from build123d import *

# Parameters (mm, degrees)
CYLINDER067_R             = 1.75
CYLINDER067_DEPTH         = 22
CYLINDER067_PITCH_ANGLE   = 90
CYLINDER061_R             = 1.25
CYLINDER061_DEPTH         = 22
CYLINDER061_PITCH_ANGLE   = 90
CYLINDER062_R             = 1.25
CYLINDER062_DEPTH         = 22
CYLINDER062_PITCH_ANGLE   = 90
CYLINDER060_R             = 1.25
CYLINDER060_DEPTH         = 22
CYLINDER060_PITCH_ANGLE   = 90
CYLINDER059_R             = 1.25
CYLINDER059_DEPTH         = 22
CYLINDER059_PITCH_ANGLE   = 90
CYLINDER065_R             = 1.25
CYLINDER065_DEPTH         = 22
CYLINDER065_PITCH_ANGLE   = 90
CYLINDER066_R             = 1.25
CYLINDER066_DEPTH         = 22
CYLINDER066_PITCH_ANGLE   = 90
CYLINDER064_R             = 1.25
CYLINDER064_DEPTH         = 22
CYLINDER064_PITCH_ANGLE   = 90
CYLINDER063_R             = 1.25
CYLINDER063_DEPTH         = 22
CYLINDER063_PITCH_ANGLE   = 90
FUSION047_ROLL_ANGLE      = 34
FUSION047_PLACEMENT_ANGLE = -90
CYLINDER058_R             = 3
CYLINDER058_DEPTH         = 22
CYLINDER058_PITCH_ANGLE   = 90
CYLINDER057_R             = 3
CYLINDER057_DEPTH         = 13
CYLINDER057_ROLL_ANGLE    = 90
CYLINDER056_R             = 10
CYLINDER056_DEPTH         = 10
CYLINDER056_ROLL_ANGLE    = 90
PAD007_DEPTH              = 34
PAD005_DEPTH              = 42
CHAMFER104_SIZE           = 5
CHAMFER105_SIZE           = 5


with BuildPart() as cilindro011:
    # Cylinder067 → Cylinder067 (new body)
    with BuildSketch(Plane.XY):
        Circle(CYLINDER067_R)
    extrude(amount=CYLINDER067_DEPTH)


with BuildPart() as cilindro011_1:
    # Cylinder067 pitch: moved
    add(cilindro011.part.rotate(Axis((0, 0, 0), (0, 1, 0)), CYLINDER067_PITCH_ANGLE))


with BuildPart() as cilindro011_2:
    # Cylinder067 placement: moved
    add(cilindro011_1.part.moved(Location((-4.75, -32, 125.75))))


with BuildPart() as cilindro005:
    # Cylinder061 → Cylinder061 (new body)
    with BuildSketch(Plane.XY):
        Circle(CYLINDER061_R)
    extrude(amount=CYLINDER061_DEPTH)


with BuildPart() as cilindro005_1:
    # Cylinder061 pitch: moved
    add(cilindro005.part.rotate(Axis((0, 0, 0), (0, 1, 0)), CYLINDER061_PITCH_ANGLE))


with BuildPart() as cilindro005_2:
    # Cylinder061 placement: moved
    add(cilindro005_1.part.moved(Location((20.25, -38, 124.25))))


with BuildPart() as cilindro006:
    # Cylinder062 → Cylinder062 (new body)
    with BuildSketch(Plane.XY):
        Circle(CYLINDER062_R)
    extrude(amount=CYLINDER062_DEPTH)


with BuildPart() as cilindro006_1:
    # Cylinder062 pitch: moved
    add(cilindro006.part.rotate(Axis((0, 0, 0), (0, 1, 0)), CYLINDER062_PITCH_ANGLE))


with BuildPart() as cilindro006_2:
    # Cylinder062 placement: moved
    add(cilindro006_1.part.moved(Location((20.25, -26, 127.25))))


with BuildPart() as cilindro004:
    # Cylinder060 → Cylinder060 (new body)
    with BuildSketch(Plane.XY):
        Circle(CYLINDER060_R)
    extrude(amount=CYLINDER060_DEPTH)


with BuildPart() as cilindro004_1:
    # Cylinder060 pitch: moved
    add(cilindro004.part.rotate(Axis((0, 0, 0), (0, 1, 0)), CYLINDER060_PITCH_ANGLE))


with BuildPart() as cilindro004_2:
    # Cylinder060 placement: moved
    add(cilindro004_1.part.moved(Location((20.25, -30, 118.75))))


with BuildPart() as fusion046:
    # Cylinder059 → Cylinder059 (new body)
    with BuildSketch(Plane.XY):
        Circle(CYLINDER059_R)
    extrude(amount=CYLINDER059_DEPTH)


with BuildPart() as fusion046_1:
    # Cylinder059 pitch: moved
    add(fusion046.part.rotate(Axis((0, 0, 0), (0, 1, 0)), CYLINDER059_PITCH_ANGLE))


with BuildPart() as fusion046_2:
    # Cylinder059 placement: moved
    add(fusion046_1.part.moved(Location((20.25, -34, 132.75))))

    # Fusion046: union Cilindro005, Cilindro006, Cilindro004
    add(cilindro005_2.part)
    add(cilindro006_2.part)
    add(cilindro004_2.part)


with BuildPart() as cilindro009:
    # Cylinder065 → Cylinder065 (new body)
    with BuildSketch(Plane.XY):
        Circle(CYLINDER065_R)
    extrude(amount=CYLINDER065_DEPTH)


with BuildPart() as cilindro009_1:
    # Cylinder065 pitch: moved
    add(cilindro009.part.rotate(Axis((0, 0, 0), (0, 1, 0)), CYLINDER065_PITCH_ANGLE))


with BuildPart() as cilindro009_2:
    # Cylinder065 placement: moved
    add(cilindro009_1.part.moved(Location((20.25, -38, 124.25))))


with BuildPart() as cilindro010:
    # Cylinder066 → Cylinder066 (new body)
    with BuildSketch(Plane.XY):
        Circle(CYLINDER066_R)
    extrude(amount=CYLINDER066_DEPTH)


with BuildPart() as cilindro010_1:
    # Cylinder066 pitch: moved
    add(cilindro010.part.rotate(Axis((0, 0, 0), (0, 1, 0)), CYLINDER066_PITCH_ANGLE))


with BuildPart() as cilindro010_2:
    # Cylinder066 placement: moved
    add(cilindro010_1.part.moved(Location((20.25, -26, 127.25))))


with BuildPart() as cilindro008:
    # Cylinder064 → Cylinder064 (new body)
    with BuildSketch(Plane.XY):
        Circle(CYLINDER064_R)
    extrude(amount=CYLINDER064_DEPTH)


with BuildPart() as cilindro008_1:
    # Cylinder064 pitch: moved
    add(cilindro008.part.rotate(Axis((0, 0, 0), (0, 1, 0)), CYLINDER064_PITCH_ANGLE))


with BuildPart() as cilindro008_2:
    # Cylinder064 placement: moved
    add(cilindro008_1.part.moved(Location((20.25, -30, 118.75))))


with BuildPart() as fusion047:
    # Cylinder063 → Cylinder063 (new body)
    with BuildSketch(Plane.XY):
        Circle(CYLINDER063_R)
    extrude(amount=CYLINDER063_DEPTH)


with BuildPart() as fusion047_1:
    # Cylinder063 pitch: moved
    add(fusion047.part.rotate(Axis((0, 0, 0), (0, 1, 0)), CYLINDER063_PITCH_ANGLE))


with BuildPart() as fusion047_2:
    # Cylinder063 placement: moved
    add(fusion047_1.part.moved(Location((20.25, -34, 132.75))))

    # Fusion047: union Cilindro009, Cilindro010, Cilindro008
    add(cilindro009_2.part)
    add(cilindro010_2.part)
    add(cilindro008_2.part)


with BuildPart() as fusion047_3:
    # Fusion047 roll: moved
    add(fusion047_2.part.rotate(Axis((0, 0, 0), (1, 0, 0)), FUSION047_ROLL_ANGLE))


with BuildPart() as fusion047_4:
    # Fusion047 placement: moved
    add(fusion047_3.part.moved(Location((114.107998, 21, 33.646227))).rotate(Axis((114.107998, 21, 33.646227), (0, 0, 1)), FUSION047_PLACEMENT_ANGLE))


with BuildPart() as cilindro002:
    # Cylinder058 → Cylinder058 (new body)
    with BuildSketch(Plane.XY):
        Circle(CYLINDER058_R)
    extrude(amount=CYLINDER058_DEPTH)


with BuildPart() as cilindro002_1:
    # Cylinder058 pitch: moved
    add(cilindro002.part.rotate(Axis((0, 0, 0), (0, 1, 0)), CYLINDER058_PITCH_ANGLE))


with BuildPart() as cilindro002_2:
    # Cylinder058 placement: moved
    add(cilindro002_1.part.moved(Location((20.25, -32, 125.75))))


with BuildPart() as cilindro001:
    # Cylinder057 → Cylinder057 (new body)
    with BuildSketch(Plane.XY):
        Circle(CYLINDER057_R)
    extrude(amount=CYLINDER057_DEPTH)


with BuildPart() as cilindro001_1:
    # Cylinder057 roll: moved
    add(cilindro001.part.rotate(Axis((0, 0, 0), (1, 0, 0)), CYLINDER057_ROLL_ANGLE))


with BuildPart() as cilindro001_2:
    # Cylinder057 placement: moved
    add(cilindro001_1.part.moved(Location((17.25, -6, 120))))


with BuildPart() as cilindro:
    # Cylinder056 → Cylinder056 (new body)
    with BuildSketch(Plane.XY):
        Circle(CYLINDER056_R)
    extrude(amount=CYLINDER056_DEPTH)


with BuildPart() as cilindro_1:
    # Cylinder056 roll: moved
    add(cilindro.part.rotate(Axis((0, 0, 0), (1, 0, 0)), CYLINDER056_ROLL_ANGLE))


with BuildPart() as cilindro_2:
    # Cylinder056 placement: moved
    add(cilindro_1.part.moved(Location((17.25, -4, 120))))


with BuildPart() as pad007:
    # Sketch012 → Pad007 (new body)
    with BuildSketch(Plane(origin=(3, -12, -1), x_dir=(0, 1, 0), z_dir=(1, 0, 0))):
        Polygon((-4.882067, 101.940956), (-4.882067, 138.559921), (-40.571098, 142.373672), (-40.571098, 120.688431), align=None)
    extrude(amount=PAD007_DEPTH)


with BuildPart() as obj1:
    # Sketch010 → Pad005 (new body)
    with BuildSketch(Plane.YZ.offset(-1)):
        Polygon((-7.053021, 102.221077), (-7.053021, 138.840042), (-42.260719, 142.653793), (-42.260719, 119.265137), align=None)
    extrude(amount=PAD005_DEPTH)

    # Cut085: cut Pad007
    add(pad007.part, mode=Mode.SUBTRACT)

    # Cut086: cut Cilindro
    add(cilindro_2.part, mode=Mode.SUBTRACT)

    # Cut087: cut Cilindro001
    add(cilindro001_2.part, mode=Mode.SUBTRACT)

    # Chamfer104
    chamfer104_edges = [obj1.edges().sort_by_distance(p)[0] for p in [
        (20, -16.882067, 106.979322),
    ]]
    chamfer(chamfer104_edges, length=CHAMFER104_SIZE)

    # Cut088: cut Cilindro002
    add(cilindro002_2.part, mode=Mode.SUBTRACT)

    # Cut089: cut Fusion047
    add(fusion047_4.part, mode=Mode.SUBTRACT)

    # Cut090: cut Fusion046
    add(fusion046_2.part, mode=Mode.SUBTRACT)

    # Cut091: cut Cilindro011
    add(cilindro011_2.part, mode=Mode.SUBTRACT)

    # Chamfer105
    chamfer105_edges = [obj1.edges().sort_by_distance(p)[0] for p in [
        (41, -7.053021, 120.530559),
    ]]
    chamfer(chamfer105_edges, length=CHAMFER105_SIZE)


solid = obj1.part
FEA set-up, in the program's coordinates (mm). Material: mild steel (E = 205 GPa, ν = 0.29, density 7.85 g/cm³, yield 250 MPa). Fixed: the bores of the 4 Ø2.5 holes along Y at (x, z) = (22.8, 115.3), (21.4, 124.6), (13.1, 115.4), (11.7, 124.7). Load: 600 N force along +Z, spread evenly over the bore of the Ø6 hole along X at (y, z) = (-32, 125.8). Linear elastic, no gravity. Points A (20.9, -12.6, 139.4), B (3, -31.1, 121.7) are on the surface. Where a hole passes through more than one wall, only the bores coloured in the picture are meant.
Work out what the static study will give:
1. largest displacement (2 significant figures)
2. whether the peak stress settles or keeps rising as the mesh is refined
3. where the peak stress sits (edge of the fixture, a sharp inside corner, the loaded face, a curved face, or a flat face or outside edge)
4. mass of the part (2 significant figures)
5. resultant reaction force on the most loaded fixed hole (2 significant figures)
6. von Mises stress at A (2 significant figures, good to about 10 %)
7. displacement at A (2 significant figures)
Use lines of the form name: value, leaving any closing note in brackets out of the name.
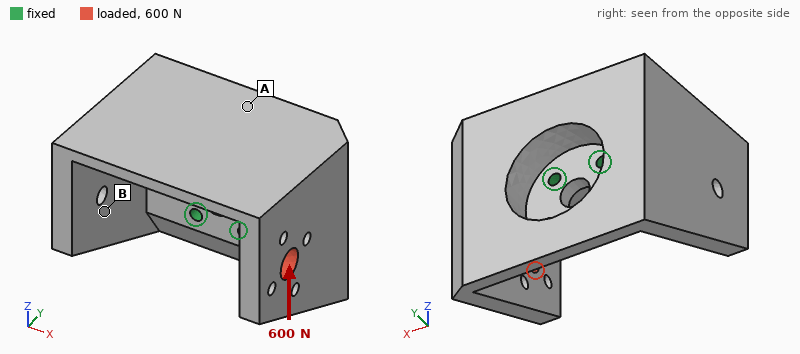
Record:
largest displacement: 28 µm
whether the peak stress settles or keeps rising as the mesh is refined: keeps rising
where the peak stress sits: edge of the fixture
mass of the part: 150 g
resultant reaction force on the most loaded fixed hole: 750 N
von Mises stress at A: 15 MPa
displacement at A: 7.5 µm
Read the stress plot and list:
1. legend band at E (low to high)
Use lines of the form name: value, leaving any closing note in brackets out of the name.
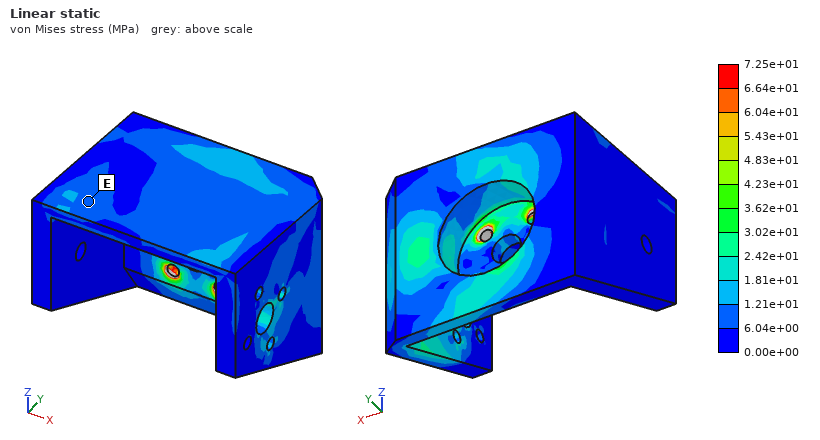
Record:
legend band at E: 6.04e+00 to 1.21e+01 MPa
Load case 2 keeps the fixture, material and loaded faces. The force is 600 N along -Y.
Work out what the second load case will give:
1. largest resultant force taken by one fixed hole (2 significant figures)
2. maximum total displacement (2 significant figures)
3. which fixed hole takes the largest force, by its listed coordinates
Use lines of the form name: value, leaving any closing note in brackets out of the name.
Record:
largest resultant force taken by one fixed hole: 780 N
maximum total displacement: 23 µm
which fixed hole takes the largest force, by its listed coordinates: (21.4, 124.6)
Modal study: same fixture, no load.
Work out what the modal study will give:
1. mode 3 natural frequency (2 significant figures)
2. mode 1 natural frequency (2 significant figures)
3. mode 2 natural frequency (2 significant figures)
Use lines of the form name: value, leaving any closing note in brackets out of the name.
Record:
mode 3 natural frequency: 7000 Hz
mode 1 natural frequency: 3500 Hz
mode 2 natural frequency: 4500 Hz
